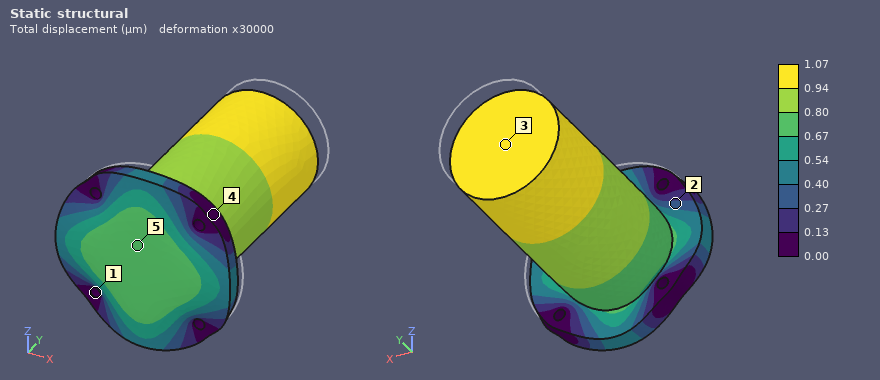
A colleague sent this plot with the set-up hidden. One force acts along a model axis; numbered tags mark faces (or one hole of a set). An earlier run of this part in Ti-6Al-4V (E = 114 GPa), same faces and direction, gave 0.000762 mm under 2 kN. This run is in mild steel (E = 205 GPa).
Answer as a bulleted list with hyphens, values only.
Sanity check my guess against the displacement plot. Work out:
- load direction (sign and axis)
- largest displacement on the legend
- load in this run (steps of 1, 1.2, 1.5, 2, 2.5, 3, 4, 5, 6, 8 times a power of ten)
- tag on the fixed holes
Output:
- -Y
- 1.07 µm
- 5 kN
- 1
